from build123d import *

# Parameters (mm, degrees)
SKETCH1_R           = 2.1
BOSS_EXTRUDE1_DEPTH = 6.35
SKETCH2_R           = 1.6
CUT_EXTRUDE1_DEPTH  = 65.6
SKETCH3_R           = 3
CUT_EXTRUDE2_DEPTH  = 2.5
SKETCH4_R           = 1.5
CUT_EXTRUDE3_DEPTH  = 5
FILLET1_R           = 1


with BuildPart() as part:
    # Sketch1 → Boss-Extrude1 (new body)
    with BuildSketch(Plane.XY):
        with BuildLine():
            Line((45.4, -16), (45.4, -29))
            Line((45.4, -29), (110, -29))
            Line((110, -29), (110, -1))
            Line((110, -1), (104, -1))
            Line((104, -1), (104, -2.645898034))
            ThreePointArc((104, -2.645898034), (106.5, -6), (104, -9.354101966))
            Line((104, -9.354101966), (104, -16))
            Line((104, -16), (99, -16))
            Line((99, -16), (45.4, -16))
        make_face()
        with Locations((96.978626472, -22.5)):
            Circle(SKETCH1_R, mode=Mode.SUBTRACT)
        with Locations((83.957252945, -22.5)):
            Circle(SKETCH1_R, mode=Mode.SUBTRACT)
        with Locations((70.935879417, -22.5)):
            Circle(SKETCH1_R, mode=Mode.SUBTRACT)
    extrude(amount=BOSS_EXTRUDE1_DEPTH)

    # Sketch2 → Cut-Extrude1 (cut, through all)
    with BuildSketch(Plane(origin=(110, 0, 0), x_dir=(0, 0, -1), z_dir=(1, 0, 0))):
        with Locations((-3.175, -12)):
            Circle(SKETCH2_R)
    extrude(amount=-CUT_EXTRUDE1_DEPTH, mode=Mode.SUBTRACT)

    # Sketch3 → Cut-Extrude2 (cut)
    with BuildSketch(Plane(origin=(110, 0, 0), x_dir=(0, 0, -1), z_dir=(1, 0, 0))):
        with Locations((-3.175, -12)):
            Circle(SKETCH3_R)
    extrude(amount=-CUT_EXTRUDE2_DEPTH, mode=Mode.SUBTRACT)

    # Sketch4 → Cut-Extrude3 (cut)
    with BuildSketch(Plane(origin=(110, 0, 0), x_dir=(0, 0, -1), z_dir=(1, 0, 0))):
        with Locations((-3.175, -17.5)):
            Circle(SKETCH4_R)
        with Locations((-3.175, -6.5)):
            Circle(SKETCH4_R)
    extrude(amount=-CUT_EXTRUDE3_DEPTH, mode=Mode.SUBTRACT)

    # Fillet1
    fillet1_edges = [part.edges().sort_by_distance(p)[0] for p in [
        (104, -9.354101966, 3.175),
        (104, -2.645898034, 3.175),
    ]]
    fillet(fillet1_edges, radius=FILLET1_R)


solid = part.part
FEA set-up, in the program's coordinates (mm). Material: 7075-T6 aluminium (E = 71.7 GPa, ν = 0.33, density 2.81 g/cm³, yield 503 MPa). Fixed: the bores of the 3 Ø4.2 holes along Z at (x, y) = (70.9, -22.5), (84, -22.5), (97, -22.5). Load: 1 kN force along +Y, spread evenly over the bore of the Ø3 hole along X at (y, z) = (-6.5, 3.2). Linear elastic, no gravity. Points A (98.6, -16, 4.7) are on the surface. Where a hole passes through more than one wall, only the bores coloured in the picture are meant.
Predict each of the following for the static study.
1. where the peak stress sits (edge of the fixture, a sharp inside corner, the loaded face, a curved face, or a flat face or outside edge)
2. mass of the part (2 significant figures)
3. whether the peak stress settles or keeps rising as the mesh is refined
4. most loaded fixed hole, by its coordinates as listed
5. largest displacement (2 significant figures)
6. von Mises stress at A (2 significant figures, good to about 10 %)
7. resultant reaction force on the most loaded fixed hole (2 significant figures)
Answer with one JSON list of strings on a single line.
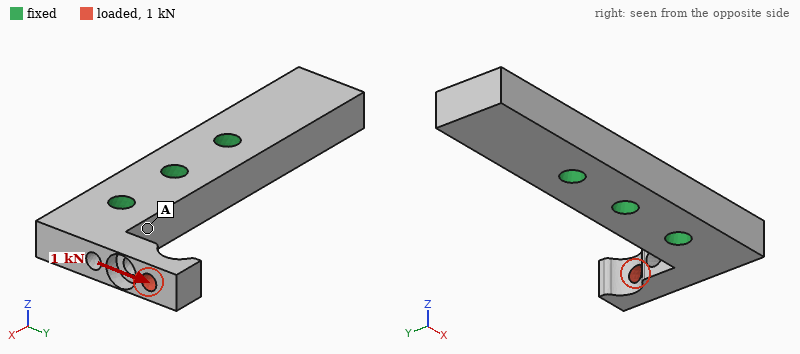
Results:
["a sharp inside corner", "15 g", "keeps rising", "(97, -22.5)", "0.14 mm", "50 MPa", "1.4 kN"]
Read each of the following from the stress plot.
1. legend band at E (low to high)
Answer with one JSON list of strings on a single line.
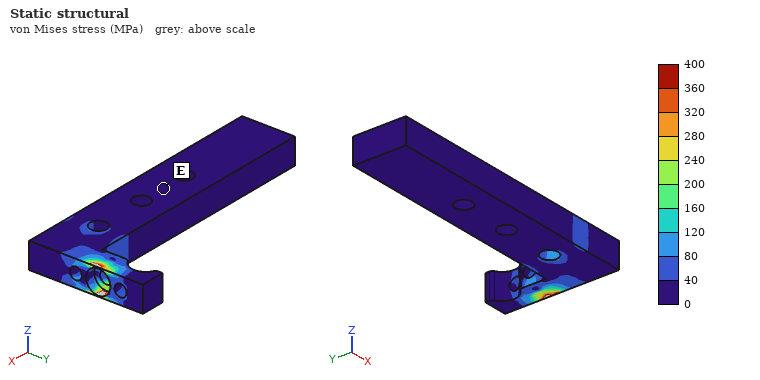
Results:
["0 to 40 MPa"]
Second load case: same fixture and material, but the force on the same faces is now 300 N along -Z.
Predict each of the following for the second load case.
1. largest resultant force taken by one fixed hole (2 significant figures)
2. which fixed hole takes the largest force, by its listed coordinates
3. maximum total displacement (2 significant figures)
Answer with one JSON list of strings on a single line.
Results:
["340 N", "(97, -22.5)", "0.13 mm"]
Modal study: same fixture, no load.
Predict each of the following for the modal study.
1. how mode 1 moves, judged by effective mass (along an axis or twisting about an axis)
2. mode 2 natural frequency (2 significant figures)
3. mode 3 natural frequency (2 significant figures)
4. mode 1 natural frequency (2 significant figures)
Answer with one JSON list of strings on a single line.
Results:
["along Z", "9600 Hz", "10000 Hz", "8000 Hz"]
